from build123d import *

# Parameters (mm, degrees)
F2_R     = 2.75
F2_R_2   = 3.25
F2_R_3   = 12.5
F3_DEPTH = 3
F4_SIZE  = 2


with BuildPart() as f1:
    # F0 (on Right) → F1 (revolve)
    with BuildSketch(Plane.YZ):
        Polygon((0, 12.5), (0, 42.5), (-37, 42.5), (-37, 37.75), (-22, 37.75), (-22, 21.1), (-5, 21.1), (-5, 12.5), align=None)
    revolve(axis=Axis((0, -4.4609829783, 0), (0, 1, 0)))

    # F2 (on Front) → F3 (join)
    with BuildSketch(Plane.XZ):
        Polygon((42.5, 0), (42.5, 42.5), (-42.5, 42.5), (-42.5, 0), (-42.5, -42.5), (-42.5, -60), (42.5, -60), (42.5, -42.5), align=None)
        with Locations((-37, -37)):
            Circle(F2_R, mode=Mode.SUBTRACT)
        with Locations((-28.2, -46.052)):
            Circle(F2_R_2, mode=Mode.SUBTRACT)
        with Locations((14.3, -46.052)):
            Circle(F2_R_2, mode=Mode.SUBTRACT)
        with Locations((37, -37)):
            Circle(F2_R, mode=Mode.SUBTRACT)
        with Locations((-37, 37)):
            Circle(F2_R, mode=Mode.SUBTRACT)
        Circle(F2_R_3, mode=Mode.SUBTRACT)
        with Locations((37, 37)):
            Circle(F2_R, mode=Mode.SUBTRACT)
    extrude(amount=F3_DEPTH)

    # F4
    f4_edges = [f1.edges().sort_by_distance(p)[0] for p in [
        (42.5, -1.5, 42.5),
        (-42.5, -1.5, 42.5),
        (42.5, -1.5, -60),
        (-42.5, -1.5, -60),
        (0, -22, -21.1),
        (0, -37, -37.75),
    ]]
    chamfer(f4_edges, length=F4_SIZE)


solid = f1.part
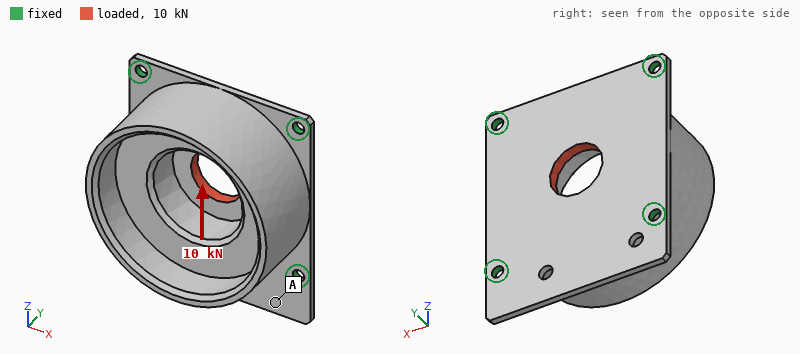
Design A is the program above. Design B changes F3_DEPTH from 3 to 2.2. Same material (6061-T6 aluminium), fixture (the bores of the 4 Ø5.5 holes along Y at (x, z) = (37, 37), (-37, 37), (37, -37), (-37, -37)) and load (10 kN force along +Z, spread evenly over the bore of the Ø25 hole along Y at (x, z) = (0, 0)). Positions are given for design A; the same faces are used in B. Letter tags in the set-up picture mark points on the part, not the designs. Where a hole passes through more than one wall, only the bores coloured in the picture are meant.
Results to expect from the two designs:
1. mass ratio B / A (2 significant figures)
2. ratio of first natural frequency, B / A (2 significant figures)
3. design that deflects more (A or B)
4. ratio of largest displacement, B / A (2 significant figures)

0.98
0.73
B
1.2
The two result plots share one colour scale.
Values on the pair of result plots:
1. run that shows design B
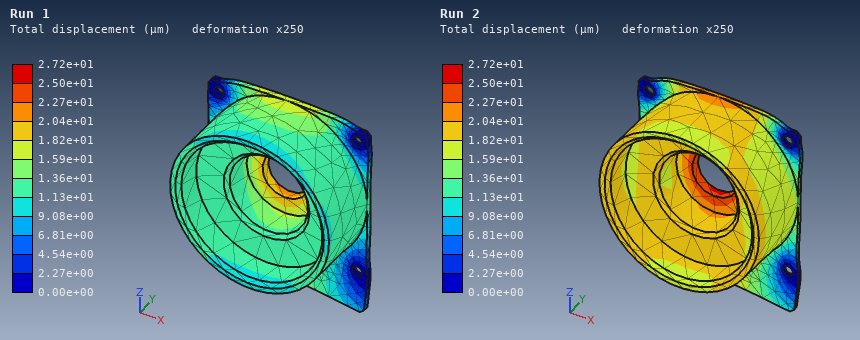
Run 2
